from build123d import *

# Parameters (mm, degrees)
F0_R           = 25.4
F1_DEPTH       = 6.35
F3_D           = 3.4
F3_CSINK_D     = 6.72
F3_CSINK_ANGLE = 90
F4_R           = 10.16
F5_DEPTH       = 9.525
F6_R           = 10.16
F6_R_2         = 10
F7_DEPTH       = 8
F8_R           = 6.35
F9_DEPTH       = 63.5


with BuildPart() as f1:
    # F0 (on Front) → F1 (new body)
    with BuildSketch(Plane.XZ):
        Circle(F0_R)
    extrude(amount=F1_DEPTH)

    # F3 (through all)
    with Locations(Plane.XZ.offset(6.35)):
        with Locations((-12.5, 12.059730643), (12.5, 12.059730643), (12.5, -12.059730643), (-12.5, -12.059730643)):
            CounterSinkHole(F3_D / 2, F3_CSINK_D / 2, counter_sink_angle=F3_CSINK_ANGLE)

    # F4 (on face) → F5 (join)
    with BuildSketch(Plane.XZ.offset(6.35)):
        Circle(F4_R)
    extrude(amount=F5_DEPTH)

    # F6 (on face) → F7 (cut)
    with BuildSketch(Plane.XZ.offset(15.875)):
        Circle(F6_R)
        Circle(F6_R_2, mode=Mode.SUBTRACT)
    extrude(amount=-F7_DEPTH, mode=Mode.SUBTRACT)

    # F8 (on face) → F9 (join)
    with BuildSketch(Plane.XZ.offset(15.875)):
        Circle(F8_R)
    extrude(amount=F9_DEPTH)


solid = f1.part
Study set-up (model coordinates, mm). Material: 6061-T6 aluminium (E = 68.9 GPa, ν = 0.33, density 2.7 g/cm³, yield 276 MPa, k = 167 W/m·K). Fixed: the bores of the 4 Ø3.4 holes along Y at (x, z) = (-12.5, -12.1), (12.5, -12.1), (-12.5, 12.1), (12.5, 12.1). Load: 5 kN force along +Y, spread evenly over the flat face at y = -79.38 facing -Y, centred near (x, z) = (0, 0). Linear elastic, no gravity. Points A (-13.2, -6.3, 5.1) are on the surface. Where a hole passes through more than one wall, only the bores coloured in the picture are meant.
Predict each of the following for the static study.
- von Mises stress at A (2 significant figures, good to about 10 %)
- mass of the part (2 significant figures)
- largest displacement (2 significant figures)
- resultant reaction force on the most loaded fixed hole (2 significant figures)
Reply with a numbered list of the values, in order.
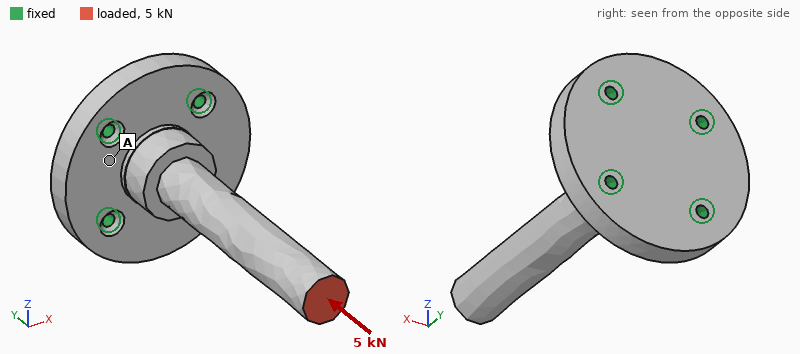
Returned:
1. 17 MPa
2. 64 g
3. 50 µm
4. 1.4 kN
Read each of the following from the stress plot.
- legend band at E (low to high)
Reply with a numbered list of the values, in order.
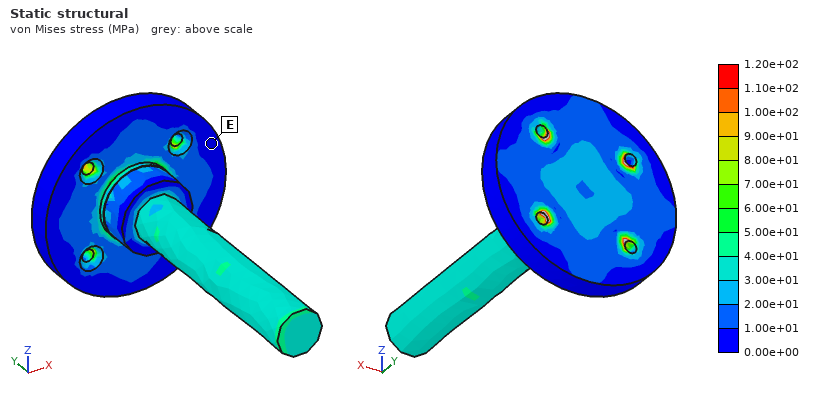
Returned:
1. 0.00e+00 to 1.00e+01 MPa
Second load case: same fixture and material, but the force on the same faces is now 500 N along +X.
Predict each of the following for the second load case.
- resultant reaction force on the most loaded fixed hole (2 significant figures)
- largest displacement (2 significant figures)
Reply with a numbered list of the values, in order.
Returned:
1. 840 N
2. 0.63 mm
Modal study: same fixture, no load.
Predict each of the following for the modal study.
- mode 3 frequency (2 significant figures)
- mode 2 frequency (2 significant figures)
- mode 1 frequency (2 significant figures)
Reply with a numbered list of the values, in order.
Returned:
1. 9900 Hz
2. 1900 Hz
3. 1900 Hz
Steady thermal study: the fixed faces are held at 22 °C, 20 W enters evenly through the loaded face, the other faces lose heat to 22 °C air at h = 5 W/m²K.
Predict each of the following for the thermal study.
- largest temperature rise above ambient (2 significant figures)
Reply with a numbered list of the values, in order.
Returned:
1. 67 K
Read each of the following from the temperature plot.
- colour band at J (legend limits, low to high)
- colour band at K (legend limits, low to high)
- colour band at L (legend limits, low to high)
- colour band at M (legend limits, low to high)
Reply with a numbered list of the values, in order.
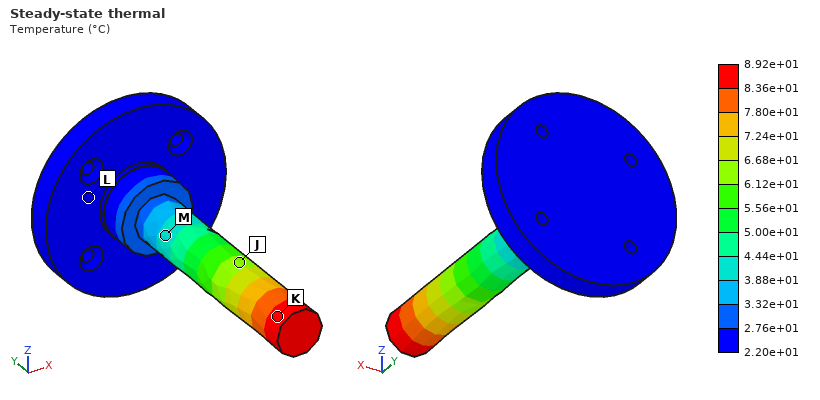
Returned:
1. 6.12e+01 to 6.68e+01 °C
2. 8.36e+01 to 8.92e+01 °C
3. 2.20e+01 to 2.76e+01 °C
4. 3.88e+01 to 4.44e+01 °C
